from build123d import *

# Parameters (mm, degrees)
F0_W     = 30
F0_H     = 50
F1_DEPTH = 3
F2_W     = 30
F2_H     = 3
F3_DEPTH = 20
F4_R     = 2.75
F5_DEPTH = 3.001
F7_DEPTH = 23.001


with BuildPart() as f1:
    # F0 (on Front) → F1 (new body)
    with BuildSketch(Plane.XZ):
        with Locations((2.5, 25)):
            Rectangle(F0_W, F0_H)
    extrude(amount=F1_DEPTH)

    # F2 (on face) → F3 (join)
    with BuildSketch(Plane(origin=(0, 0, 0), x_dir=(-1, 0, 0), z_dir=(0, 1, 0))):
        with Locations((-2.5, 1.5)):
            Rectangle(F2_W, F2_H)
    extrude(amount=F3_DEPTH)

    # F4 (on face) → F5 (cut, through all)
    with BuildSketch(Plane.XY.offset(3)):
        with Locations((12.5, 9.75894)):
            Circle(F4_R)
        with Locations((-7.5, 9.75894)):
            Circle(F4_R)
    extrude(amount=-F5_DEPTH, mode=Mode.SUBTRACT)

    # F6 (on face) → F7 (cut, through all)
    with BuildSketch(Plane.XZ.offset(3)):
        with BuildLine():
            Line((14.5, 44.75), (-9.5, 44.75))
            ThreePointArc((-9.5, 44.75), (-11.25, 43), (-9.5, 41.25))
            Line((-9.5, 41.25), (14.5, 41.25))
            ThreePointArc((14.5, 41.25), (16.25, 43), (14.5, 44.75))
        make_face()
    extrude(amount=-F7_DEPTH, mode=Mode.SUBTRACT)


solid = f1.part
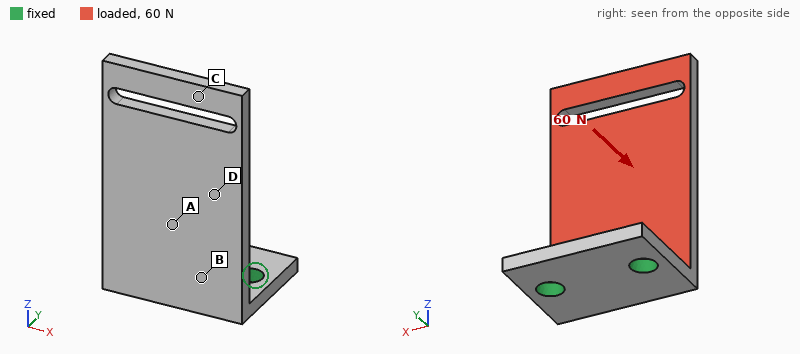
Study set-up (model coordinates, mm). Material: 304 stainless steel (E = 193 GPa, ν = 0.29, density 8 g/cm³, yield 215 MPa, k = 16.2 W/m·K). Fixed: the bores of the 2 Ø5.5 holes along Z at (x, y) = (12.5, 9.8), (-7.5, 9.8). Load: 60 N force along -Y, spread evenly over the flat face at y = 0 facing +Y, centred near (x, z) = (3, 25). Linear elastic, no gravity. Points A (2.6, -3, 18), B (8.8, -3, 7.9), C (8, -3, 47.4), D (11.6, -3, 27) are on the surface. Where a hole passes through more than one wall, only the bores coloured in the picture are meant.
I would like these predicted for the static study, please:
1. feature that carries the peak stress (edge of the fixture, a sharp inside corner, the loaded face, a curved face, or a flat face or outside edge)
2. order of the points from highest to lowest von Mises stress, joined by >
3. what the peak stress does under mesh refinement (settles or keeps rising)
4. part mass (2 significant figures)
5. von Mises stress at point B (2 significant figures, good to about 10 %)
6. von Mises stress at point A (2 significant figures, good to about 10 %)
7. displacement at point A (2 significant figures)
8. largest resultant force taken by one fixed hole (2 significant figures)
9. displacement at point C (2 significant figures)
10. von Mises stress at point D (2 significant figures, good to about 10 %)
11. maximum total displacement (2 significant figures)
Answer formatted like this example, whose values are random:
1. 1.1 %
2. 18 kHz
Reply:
1. edge of the fixture
2. B > A > D > C
3. keeps rising
4. 47 g
5. 21 MPa
6. 12 MPa
7. 0.028 mm
8. 32 N
9. 0.100 mm
10. 6.6 MPa
11. 0.11 mm
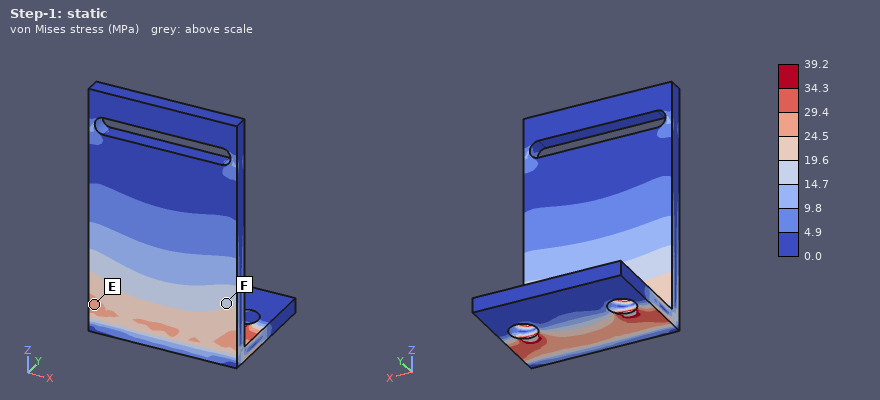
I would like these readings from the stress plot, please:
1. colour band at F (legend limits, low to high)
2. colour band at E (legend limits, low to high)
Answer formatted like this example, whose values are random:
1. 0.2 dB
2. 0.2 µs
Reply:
1. 14.7 to 19.6 MPa
2. 24.5 to 29.4 MPa
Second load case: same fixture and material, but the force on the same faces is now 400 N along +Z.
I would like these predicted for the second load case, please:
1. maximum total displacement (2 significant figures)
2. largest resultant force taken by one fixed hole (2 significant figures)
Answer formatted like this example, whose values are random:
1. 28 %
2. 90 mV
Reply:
1. 19 µm
2. 200 N
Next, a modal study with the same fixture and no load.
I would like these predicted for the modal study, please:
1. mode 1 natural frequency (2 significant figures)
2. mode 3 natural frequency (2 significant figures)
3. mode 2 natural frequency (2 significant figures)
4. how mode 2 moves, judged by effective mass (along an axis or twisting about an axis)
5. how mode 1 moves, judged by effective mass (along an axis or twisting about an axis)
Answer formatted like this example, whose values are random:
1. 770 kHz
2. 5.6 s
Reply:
1. 850 Hz
2. 3700 Hz
3. 2600 Hz
4. along X
5. along Y
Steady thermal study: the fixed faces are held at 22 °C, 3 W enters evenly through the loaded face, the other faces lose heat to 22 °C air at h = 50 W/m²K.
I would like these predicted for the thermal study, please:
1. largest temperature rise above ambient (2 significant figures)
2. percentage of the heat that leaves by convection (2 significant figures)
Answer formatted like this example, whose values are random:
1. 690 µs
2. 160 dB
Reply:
1. 22 K
2. 64 %
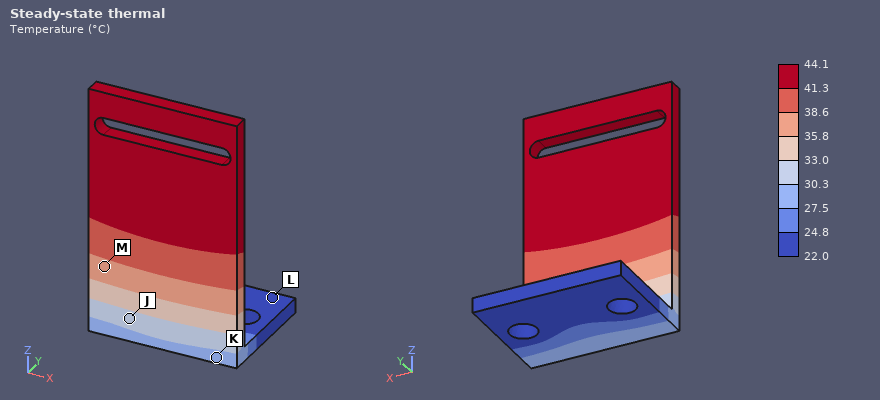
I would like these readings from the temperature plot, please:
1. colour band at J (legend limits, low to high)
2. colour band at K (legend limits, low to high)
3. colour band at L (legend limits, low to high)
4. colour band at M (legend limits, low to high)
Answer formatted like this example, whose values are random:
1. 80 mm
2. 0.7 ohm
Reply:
1. 30.3 to 33.0 °C
2. 27.5 to 30.3 °C
3. 22.0 to 24.8 °C
4. 35.8 to 38.6 °C
